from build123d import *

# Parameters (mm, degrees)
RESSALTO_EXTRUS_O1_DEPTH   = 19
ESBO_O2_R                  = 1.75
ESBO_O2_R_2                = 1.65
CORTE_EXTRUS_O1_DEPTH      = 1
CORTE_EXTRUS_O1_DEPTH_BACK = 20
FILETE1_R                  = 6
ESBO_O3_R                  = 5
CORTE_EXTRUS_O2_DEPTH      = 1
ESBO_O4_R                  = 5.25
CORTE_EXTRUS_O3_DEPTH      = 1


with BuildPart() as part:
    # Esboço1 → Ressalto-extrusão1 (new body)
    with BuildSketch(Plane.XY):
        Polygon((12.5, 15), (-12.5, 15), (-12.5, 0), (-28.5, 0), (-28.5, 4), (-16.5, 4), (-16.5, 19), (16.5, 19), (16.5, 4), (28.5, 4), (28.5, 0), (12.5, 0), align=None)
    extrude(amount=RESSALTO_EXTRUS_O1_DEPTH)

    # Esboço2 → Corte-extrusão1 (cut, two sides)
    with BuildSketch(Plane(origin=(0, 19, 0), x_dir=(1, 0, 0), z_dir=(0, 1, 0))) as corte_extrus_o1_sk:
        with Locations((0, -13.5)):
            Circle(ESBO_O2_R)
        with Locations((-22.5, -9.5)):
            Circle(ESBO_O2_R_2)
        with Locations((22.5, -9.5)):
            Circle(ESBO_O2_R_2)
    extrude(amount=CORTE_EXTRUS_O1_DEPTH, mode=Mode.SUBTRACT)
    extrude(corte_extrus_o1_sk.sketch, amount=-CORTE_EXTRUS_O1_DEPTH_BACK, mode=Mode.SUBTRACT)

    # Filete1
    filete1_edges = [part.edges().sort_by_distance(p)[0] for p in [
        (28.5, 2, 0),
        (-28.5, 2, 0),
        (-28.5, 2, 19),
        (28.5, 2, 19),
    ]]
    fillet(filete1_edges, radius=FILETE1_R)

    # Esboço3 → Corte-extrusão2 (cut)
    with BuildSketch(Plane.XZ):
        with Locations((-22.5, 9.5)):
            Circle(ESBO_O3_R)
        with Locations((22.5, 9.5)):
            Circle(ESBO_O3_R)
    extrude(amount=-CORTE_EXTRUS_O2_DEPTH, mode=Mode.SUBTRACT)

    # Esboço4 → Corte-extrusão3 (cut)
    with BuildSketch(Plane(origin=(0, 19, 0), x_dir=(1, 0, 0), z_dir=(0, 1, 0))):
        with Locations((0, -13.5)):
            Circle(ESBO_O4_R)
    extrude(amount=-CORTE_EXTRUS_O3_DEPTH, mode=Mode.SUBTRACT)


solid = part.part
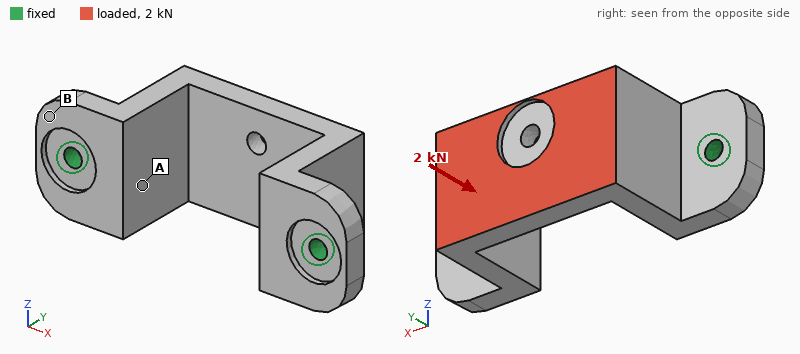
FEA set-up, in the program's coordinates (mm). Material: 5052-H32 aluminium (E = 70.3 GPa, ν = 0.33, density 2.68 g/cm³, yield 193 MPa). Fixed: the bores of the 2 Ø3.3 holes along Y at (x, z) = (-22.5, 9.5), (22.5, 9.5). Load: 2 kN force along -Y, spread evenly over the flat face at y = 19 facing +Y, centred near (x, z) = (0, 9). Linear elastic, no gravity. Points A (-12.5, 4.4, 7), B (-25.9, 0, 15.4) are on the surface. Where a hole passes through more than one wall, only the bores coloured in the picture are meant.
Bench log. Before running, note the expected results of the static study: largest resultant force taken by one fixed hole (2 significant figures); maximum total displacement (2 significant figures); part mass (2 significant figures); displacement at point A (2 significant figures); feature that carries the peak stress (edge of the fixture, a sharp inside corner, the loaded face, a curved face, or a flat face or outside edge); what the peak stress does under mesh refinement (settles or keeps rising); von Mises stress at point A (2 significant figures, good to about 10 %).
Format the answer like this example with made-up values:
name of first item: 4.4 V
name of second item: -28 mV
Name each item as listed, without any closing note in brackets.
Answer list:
largest resultant force taken by one fixed hole: 1.1 kN
maximum total displacement: 57 µm
part mass: 17 g
displacement at point A: 25 µm
feature that carries the peak stress: edge of the fixture
what the peak stress does under mesh refinement: keeps rising
von Mises stress at point A: 35 MPa
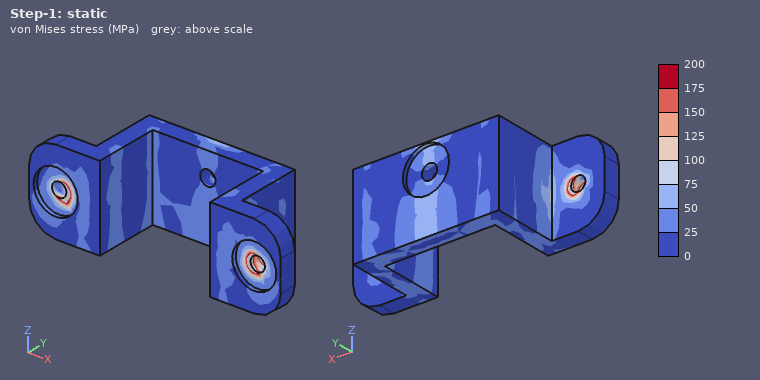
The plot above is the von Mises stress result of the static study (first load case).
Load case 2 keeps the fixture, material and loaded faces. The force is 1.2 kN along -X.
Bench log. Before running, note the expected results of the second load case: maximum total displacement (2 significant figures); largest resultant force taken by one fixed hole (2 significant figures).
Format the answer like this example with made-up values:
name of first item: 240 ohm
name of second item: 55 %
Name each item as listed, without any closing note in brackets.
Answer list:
maximum total displacement: 64 µm
largest resultant force taken by one fixed hole: 730 N
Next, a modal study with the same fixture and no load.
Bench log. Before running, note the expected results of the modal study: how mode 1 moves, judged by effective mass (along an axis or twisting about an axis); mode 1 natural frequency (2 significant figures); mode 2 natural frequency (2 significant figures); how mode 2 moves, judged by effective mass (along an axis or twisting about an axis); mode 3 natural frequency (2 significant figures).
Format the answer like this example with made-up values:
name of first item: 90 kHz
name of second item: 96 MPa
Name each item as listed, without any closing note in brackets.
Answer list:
how mode 1 moves, judged by effective mass: along Z
mode 1 natural frequency: 4500 Hz
mode 2 natural frequency: 7700 Hz
how mode 2 moves, judged by effective mass: along X
mode 3 natural frequency: 9200 Hz
